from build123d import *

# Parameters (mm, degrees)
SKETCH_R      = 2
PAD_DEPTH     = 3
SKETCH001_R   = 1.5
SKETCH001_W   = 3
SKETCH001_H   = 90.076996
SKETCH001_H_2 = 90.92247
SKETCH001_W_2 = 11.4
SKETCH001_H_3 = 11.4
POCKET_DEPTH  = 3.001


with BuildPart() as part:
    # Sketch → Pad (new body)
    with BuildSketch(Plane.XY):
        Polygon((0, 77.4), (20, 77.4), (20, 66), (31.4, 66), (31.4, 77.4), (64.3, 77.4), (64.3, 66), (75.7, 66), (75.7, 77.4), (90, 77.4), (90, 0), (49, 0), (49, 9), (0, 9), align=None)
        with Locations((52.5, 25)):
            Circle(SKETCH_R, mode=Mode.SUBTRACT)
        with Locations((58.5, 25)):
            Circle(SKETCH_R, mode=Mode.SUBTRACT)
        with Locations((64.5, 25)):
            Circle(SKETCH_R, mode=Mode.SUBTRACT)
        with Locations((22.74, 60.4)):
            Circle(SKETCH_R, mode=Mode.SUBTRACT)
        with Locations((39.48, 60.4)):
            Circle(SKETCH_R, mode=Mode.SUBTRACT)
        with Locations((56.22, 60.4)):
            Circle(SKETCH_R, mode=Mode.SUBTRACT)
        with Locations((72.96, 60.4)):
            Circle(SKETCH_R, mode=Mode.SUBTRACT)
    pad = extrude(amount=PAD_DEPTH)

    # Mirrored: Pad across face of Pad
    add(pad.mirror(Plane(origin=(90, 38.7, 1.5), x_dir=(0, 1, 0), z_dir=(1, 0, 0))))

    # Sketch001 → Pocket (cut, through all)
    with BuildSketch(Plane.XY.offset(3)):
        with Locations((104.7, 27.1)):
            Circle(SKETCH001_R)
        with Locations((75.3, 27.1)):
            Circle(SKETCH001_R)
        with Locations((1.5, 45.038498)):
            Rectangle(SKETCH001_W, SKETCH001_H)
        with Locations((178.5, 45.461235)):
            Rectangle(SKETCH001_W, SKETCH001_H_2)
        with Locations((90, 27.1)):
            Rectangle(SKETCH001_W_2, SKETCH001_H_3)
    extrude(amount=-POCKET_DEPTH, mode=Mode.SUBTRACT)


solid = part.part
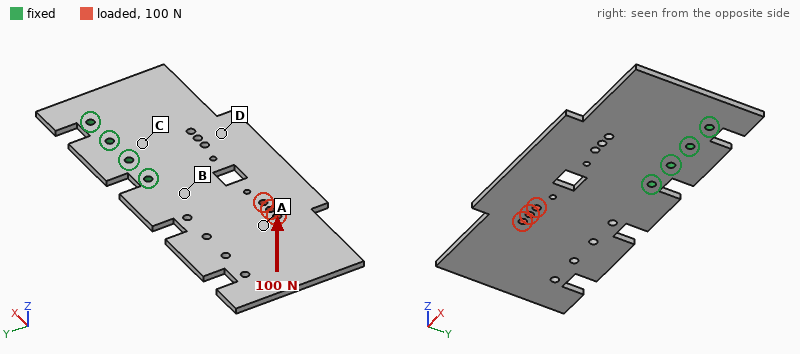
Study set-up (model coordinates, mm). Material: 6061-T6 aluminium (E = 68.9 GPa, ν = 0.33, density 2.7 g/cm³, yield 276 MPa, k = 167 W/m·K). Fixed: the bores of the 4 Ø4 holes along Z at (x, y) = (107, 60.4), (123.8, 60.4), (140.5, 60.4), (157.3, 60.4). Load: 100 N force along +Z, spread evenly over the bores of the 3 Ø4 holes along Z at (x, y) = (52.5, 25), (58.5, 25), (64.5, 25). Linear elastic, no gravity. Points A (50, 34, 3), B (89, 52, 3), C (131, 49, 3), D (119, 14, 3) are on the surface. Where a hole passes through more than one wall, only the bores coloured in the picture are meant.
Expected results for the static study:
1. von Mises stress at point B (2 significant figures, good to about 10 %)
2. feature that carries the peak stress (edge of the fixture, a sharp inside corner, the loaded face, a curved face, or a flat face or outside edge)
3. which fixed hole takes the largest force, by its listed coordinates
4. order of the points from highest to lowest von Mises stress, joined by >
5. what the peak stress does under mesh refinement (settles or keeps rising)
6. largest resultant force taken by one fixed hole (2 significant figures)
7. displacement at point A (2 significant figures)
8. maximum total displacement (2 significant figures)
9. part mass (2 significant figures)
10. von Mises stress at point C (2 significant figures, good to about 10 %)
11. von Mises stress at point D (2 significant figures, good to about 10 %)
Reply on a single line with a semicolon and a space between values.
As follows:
38 MPa; edge of the fixture; (107, 60.4); B > D > C > A; keeps rising; 200 N; 0.90 mm; 2.0 mm; 96 g; 15 MPa; 26 MPa
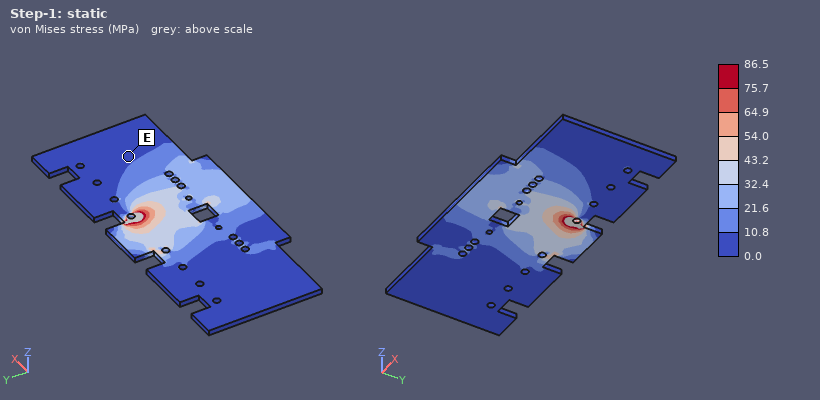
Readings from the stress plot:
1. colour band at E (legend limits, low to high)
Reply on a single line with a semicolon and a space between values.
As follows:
0.0 to 10.8 MPa
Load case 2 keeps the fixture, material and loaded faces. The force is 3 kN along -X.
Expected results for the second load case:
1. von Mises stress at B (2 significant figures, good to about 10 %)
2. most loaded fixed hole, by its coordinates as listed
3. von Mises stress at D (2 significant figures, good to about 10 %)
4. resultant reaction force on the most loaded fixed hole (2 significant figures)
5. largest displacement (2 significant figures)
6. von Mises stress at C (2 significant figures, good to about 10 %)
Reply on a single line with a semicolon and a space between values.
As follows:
9.1 MPa; (107, 60.4); 27 MPa; 2.1 kN; 0.16 mm; 33 MPa
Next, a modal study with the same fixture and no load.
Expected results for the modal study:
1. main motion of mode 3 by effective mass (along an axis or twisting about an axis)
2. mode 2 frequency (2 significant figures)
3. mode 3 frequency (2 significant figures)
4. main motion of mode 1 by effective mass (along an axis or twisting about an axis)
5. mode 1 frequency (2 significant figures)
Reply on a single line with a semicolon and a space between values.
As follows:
along Z; 490 Hz; 960 Hz; along Z; 190 Hz
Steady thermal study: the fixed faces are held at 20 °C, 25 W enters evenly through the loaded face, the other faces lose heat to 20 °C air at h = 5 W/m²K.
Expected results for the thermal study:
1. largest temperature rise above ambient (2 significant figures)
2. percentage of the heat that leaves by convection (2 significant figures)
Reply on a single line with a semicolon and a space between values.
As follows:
59 K; 13 %
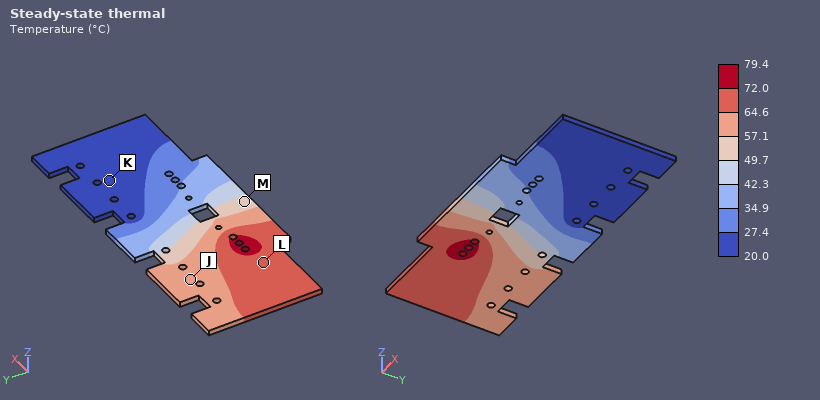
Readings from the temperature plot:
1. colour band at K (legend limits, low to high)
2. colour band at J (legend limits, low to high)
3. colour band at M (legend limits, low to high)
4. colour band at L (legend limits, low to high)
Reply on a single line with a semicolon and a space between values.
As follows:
20.0 to 27.4 °C; 57.1 to 64.6 °C; 49.7 to 57.1 °C; 64.6 to 72.0 °C
